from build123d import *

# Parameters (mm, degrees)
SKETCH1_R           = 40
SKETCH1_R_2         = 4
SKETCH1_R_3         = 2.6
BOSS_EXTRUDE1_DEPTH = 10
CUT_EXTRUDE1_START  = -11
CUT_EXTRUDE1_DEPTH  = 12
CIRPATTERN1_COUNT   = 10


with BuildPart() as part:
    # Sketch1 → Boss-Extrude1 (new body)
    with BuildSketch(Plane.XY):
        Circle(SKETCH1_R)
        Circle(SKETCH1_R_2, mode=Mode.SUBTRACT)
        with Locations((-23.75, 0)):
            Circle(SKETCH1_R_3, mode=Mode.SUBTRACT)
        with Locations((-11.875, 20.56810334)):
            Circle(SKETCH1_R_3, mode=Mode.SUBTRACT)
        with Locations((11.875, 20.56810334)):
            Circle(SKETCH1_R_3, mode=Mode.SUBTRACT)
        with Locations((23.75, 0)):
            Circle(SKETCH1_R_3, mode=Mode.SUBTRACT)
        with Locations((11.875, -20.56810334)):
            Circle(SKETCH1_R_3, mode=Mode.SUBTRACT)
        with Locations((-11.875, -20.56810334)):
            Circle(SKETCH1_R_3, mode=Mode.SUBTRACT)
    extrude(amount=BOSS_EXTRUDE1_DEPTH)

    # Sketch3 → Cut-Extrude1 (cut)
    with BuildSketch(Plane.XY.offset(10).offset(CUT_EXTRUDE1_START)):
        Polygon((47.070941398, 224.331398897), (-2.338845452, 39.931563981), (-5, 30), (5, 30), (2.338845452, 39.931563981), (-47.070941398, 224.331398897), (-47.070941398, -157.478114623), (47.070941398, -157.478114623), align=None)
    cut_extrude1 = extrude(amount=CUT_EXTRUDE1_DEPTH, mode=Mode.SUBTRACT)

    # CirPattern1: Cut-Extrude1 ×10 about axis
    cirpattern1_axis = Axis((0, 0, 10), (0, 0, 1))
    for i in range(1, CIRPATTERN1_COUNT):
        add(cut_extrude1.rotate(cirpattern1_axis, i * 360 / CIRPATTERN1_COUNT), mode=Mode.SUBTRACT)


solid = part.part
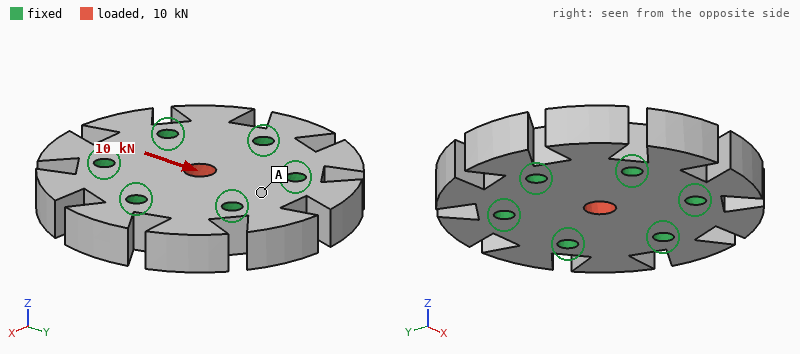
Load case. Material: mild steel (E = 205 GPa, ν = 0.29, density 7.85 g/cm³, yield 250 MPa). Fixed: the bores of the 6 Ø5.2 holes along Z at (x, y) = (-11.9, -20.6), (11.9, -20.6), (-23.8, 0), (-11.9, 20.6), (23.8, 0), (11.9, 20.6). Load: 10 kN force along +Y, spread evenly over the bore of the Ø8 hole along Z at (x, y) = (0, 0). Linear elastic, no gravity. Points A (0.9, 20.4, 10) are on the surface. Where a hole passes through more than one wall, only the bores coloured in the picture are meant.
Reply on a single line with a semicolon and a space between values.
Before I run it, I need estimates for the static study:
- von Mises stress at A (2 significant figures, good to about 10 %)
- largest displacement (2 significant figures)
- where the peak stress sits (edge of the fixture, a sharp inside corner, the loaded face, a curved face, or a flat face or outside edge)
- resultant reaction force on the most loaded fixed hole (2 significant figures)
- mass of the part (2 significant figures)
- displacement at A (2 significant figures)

6.3 MPa; 2.5 µm; the loaded face; 2.3 kN; 320 g; 0.76 µm
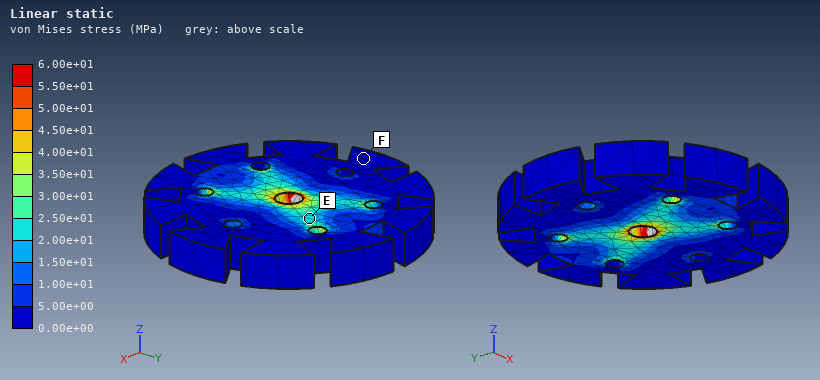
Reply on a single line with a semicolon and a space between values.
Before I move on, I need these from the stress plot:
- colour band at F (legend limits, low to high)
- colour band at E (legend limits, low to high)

0.00e+00 to 5.00e+00 MPa; 2.00e+01 to 2.50e+01 MPa
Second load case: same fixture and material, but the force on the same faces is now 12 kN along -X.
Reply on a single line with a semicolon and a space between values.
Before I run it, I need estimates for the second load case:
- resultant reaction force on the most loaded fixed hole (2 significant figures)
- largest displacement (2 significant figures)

3.2 kN; 2.9 µm
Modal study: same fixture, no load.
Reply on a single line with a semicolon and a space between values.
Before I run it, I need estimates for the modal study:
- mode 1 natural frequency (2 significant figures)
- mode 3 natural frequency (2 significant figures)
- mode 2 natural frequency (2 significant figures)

18 kHz; 18 kHz; 18 kHz
